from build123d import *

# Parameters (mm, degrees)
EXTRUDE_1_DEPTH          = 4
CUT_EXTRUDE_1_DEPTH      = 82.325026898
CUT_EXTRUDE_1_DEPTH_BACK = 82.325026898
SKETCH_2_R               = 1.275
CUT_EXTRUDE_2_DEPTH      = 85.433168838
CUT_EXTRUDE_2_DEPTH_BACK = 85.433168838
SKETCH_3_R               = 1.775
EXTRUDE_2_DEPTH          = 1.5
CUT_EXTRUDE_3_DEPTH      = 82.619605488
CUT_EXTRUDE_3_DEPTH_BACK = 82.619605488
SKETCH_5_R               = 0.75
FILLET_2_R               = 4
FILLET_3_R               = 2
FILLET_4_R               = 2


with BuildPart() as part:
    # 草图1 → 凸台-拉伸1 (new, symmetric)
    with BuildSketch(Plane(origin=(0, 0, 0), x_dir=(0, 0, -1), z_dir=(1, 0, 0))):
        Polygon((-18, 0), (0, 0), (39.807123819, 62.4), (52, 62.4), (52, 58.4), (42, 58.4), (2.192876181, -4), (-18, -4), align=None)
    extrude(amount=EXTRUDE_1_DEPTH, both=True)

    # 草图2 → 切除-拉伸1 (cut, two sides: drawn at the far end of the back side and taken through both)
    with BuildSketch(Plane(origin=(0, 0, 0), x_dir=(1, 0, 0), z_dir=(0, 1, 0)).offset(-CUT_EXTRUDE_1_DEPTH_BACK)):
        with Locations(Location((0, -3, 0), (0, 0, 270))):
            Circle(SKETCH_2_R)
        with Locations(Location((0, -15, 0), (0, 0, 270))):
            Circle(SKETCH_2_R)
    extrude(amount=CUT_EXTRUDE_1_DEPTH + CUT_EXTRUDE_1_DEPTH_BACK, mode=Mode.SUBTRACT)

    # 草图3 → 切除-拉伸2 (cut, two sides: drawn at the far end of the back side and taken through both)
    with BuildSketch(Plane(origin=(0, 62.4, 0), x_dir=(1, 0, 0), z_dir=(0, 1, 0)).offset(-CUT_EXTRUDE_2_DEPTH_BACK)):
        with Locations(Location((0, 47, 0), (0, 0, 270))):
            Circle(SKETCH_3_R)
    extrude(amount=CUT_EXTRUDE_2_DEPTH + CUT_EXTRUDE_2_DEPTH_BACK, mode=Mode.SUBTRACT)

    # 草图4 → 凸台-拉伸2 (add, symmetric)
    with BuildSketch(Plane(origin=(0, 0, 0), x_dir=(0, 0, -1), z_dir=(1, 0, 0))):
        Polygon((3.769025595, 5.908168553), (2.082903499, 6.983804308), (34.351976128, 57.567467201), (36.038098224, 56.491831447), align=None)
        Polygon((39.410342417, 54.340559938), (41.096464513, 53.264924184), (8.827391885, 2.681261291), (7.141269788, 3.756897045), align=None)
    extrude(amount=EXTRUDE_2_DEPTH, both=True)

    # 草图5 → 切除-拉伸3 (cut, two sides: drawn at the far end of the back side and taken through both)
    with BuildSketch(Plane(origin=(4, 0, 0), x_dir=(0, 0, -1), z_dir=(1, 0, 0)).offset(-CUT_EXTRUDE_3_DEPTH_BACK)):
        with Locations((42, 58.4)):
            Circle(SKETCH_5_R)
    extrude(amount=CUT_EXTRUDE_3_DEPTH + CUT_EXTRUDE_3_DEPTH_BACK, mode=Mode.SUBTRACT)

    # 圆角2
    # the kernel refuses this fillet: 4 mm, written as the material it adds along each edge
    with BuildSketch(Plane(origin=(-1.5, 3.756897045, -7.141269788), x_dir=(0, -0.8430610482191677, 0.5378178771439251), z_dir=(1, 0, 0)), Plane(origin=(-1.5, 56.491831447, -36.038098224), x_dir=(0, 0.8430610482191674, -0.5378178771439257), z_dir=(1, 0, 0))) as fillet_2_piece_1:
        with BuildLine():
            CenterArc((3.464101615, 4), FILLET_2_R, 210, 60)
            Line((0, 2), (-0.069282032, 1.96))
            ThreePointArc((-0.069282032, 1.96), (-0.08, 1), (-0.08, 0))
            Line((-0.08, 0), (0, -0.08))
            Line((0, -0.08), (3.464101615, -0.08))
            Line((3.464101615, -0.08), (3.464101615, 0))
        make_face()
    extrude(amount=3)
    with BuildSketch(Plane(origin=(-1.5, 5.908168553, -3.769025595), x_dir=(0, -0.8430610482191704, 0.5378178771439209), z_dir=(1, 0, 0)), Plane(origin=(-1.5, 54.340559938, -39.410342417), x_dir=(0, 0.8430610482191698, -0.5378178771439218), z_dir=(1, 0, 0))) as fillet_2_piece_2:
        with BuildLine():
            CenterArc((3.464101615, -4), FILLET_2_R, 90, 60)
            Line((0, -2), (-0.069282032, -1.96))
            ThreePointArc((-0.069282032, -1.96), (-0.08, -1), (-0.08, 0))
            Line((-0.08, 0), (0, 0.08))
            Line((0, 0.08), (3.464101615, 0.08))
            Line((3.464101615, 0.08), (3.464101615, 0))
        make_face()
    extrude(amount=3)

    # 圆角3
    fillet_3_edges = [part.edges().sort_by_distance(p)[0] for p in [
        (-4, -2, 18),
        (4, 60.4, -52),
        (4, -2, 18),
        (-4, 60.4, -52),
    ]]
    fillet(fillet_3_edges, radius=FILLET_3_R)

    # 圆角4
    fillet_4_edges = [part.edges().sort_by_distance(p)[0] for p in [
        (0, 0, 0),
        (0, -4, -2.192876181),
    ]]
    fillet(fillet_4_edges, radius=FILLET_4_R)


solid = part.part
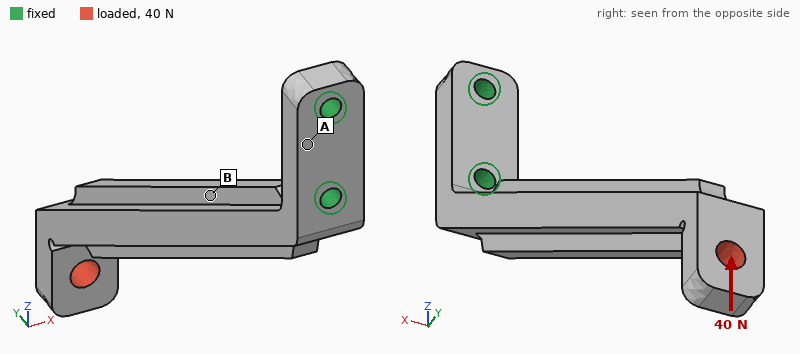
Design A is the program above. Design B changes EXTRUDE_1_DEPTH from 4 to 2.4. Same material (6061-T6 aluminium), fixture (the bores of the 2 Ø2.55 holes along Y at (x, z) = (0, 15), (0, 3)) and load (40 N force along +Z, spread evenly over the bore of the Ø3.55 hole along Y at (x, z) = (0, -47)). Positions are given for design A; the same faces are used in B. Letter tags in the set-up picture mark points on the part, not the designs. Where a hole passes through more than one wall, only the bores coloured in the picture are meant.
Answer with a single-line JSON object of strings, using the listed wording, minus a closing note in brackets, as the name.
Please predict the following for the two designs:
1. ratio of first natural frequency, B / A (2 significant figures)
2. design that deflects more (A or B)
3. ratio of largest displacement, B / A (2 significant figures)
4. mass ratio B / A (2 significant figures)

{"ratio of first natural frequency, B / A": "0.91", "design that deflects more": "B", "ratio of largest displacement, B / A": "1.4", "mass ratio B / A": "0.67"}
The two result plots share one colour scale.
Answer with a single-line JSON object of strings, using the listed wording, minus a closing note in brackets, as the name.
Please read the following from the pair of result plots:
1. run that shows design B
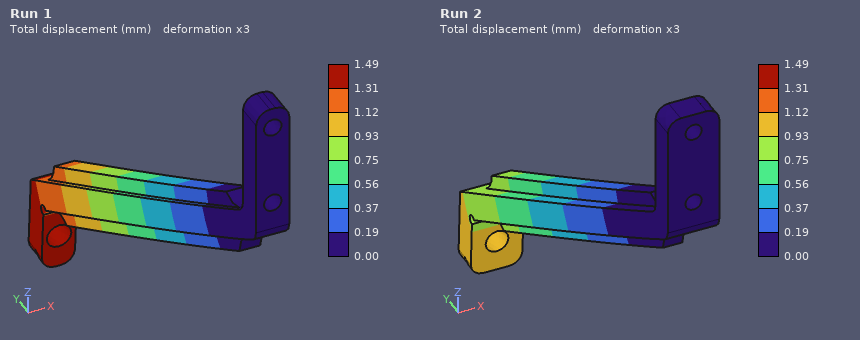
{"run that shows design B": "Run 1"}
